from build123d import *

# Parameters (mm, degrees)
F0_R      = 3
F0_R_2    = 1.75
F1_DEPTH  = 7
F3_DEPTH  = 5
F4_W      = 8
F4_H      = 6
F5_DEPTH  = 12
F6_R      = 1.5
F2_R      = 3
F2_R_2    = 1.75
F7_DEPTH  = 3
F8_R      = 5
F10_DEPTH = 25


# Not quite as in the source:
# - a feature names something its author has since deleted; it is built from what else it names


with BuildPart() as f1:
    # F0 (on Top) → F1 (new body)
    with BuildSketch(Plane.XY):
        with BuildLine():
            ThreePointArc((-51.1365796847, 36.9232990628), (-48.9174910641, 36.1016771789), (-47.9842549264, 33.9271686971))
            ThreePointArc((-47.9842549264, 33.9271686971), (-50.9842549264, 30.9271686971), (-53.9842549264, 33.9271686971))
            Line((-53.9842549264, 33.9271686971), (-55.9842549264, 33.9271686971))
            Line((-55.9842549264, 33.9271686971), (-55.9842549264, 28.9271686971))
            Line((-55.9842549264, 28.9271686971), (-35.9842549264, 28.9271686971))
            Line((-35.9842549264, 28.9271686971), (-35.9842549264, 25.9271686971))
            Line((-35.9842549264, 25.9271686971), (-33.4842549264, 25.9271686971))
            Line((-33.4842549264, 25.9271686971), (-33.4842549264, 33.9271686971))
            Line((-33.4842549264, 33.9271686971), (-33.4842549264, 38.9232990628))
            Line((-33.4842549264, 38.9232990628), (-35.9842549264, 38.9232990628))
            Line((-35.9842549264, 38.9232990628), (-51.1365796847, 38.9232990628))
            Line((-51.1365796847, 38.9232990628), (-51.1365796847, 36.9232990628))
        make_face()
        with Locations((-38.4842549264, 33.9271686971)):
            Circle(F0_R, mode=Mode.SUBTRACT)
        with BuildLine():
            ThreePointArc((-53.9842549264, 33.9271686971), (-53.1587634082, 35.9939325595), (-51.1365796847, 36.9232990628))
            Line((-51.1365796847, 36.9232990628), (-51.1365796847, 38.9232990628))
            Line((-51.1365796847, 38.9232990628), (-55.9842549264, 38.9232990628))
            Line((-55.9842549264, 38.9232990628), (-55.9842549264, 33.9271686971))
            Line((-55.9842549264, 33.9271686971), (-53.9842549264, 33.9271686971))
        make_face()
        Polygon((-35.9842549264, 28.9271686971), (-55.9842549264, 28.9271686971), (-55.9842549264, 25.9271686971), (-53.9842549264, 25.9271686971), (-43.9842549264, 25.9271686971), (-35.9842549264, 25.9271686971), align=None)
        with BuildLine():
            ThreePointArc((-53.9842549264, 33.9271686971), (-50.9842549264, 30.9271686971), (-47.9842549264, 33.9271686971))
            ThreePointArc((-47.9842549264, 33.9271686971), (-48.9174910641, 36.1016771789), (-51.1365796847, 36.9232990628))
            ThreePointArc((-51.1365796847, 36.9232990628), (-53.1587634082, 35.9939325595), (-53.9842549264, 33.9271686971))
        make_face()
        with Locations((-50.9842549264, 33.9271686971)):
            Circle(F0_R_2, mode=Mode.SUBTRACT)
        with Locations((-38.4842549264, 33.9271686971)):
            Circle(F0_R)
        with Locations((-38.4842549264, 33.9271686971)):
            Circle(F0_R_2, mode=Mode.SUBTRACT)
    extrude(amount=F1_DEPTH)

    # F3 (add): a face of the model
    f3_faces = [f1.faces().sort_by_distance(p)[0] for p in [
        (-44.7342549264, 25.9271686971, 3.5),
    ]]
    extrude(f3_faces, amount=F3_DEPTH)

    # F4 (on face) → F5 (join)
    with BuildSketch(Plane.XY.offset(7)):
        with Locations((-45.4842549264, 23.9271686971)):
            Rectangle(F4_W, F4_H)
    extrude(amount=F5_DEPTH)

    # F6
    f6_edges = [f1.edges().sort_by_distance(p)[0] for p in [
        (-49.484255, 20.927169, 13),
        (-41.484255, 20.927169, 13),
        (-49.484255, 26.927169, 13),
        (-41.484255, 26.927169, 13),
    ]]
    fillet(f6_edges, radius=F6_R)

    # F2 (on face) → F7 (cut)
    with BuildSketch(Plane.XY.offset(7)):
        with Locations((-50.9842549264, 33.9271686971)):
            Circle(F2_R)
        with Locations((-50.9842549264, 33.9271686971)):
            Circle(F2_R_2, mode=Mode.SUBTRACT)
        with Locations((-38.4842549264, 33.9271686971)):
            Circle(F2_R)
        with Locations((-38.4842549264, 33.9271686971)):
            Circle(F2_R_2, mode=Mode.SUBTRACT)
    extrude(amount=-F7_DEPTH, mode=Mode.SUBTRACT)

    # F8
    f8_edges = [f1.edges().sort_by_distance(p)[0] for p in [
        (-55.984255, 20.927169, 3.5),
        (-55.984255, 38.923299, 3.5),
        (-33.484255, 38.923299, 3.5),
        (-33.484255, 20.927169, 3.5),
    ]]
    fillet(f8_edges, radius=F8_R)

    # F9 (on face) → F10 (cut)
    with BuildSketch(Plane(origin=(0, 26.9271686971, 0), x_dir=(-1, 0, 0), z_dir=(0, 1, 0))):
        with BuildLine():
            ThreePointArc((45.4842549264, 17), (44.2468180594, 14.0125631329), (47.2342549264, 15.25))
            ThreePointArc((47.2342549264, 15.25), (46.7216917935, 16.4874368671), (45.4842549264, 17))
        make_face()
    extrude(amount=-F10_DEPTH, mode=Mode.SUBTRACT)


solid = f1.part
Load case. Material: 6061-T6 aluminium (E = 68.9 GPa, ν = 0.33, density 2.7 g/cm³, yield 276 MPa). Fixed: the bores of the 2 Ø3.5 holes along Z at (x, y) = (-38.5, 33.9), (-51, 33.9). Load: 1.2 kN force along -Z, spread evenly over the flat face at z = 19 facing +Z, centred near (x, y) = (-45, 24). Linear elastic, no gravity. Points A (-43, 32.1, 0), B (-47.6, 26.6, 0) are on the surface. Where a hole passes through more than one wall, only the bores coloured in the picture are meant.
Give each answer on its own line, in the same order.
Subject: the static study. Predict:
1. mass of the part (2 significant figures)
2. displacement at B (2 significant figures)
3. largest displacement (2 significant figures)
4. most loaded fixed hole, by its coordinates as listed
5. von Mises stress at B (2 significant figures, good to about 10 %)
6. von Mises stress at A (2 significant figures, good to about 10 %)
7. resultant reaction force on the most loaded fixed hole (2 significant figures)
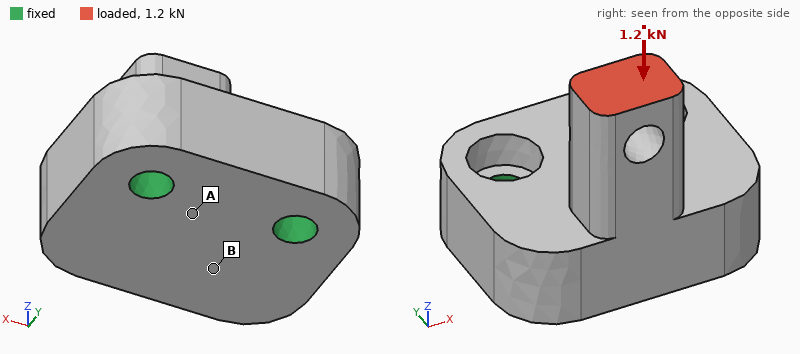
7.9 g
20 µm
72 µm
(-51, 33.9)
25 MPa
44 MPa
670 N
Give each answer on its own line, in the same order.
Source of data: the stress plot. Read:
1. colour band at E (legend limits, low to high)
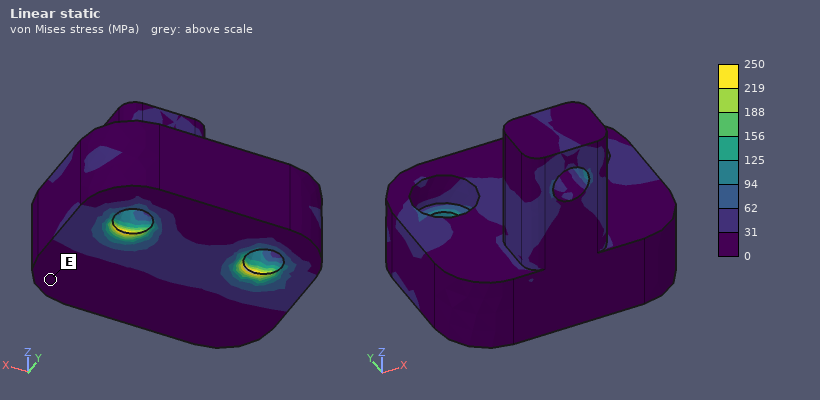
0 to 31 MPa
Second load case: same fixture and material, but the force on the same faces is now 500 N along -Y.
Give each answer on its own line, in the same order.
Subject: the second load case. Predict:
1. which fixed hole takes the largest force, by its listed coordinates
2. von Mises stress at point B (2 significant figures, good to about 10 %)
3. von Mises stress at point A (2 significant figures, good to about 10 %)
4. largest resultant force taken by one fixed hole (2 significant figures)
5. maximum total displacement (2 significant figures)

(-51, 33.9)
39 MPa
37 MPa
280 N
0.12 mm
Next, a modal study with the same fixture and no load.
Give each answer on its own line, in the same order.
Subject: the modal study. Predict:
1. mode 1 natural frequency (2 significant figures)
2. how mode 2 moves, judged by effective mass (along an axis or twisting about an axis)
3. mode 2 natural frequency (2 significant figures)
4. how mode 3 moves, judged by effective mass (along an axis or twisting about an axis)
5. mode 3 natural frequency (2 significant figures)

12 kHz
along X
20 kHz
along Z
27 kHz
